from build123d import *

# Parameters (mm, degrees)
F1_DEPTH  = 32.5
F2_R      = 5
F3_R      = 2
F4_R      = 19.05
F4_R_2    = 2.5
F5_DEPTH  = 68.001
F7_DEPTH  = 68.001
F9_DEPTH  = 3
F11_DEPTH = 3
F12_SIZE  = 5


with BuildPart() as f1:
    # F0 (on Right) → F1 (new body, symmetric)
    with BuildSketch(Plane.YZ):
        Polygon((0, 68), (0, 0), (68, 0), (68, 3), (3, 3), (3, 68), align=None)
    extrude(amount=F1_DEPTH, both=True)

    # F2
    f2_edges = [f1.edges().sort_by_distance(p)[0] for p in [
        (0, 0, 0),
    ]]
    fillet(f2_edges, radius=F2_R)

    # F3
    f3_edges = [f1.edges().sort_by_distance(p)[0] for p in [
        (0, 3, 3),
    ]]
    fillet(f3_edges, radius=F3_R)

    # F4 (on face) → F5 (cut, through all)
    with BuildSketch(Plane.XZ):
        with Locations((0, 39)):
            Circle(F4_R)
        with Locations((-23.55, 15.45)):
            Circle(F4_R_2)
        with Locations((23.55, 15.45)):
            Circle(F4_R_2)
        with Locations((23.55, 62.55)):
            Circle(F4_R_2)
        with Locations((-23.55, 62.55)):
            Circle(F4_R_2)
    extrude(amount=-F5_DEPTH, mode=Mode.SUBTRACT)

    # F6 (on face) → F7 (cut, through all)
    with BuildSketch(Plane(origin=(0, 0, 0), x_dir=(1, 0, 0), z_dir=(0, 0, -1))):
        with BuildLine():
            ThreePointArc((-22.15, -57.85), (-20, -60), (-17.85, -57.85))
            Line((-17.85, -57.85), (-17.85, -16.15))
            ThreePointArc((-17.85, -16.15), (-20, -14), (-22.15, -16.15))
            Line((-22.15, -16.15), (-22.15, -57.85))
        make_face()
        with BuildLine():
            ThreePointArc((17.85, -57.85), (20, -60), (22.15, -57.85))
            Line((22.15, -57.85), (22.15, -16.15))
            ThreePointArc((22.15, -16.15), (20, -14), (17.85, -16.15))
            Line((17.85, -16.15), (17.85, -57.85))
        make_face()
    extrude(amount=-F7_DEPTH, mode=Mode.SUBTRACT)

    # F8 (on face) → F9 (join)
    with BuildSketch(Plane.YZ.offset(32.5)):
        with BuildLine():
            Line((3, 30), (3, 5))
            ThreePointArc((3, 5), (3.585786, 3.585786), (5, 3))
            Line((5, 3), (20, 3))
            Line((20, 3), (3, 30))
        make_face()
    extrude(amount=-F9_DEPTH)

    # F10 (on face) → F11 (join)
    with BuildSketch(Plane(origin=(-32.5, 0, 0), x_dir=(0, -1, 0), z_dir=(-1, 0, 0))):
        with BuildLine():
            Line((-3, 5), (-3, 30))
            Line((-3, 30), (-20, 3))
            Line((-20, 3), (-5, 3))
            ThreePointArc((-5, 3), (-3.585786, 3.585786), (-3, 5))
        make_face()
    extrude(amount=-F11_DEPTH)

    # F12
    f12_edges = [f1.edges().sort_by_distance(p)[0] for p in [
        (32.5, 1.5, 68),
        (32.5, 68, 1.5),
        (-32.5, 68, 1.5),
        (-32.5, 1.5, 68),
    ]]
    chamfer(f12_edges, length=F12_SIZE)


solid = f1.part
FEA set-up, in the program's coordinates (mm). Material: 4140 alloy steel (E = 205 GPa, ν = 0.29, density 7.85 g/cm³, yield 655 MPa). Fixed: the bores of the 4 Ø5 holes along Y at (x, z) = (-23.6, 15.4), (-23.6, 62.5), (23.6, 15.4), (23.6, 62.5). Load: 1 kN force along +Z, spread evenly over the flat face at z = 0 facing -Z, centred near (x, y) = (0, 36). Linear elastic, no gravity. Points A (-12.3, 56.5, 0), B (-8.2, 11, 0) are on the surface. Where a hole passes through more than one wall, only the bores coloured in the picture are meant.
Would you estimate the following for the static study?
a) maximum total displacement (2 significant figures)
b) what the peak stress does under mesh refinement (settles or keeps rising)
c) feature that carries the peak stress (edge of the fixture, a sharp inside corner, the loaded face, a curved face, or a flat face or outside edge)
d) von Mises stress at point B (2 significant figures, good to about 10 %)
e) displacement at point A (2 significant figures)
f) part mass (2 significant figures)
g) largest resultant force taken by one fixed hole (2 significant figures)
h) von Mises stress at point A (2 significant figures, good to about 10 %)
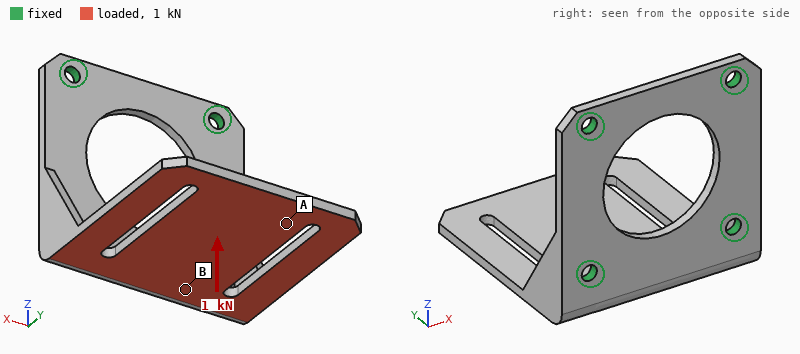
1.2 mm
keeps rising
edge of the fixture
150 MPa
0.91 mm
170 g
540 N
58 MPa
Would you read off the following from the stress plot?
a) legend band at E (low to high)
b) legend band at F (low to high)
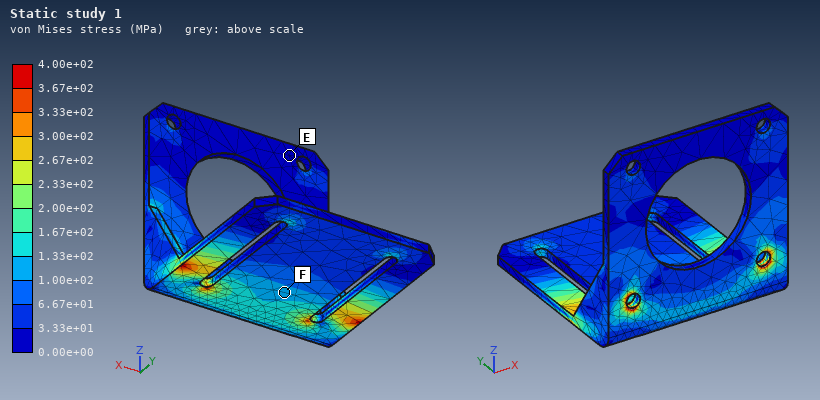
0.00e+00 to 3.33e+01 MPa
1.00e+02 to 1.33e+02 MPa
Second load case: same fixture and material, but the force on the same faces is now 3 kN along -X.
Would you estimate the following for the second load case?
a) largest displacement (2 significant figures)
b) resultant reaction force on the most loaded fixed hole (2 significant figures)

0.21 mm
2.7 kN
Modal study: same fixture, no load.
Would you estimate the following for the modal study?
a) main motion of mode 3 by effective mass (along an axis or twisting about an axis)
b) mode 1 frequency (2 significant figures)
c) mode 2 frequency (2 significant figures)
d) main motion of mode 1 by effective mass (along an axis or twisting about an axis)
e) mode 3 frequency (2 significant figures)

along X
620 Hz
1600 Hz
along Z
2500 Hz
